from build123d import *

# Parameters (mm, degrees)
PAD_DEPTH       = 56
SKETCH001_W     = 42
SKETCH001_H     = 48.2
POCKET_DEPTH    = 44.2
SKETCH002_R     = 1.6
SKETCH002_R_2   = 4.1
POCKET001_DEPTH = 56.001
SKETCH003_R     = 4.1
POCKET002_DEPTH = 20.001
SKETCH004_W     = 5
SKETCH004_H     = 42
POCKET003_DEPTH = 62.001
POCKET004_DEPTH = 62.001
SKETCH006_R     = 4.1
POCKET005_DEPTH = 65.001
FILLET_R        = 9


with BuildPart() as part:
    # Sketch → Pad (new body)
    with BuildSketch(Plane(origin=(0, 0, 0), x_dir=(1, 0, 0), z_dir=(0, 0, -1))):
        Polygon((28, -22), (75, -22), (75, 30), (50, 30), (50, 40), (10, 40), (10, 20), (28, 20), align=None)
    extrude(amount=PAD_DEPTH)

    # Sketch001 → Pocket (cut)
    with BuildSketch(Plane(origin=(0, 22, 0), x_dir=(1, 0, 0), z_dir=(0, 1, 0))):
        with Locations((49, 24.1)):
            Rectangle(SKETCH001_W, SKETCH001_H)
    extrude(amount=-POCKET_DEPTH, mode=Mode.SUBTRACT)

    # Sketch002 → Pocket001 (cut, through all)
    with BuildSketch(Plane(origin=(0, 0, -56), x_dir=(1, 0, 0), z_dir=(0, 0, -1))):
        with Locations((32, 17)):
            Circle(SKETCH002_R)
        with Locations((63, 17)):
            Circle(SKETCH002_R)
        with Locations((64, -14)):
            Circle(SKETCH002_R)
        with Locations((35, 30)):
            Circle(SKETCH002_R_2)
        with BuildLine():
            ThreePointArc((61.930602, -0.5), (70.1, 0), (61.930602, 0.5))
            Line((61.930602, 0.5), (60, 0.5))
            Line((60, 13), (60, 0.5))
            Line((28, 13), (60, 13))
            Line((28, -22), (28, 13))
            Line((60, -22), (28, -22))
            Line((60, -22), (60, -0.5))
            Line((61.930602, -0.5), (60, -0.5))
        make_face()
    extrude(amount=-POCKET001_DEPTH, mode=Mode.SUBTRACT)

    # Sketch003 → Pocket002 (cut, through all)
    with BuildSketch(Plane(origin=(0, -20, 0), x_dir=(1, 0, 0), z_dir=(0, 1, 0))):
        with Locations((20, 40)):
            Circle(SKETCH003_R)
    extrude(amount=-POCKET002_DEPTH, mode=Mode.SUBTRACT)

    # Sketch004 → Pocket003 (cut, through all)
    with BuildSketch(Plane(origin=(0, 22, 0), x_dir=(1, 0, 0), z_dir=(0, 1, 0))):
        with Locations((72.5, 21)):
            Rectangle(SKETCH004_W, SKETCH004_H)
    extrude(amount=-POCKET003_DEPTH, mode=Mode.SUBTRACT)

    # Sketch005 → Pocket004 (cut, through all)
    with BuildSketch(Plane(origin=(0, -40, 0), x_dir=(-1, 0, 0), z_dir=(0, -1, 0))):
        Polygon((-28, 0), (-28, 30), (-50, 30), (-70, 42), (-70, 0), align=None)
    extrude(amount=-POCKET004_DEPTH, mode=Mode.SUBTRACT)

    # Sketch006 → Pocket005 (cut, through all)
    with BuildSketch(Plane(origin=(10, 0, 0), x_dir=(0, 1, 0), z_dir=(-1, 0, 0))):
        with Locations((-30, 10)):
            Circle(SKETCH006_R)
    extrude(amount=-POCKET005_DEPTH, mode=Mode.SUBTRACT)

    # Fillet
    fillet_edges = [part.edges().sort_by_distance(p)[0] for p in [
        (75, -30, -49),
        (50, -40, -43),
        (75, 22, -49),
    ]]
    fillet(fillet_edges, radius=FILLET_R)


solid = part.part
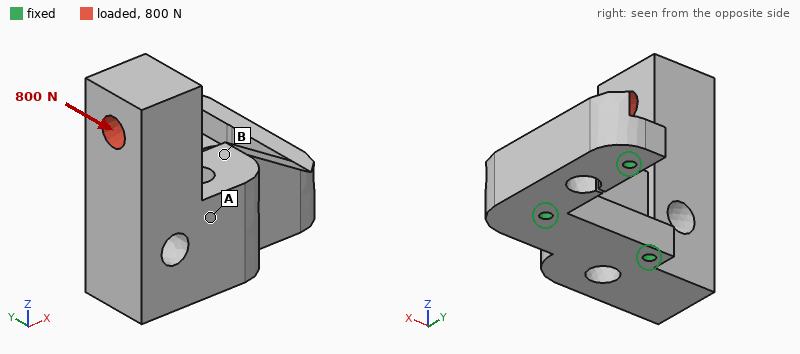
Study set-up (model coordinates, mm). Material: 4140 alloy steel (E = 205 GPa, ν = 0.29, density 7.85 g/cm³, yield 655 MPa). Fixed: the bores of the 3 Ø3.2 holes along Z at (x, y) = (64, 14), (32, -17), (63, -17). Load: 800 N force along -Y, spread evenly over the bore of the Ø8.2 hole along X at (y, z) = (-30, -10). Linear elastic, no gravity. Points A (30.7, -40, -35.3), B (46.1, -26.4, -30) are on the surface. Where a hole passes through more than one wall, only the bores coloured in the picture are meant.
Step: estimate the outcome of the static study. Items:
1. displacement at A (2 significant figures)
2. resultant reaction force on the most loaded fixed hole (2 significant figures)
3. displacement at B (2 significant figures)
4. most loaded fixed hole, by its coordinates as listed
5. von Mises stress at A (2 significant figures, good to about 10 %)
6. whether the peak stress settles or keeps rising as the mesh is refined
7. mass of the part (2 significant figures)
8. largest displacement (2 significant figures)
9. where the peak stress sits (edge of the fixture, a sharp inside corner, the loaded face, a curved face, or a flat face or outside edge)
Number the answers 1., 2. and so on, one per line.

1. 0.041 mm
2. 1.2 kN
3. 0.031 mm
4. (32, -17)
5. 31 MPa
6. keeps rising
7. 300 g
8. 0.10 mm
9. edge of the fixture
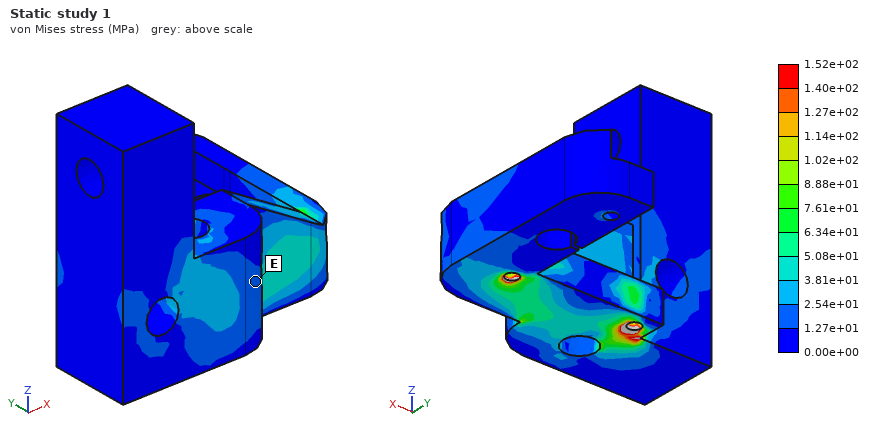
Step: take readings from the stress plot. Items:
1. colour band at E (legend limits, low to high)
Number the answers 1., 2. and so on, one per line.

1. 1.27e+01 to 2.54e+01 MPa
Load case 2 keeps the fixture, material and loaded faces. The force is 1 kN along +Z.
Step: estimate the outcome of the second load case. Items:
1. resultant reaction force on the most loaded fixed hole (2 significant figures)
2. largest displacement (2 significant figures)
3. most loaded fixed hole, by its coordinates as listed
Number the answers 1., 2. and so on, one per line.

1. 1.3 kN
2. 31 µm
3. (32, -17)
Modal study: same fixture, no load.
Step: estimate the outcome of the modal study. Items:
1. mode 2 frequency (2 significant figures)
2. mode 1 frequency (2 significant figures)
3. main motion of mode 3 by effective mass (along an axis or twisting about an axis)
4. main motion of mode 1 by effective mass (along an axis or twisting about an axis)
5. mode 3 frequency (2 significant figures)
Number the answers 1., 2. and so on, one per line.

1. 3800 Hz
2. 1800 Hz
3. along Z
4. along Y
5. 8100 Hz
